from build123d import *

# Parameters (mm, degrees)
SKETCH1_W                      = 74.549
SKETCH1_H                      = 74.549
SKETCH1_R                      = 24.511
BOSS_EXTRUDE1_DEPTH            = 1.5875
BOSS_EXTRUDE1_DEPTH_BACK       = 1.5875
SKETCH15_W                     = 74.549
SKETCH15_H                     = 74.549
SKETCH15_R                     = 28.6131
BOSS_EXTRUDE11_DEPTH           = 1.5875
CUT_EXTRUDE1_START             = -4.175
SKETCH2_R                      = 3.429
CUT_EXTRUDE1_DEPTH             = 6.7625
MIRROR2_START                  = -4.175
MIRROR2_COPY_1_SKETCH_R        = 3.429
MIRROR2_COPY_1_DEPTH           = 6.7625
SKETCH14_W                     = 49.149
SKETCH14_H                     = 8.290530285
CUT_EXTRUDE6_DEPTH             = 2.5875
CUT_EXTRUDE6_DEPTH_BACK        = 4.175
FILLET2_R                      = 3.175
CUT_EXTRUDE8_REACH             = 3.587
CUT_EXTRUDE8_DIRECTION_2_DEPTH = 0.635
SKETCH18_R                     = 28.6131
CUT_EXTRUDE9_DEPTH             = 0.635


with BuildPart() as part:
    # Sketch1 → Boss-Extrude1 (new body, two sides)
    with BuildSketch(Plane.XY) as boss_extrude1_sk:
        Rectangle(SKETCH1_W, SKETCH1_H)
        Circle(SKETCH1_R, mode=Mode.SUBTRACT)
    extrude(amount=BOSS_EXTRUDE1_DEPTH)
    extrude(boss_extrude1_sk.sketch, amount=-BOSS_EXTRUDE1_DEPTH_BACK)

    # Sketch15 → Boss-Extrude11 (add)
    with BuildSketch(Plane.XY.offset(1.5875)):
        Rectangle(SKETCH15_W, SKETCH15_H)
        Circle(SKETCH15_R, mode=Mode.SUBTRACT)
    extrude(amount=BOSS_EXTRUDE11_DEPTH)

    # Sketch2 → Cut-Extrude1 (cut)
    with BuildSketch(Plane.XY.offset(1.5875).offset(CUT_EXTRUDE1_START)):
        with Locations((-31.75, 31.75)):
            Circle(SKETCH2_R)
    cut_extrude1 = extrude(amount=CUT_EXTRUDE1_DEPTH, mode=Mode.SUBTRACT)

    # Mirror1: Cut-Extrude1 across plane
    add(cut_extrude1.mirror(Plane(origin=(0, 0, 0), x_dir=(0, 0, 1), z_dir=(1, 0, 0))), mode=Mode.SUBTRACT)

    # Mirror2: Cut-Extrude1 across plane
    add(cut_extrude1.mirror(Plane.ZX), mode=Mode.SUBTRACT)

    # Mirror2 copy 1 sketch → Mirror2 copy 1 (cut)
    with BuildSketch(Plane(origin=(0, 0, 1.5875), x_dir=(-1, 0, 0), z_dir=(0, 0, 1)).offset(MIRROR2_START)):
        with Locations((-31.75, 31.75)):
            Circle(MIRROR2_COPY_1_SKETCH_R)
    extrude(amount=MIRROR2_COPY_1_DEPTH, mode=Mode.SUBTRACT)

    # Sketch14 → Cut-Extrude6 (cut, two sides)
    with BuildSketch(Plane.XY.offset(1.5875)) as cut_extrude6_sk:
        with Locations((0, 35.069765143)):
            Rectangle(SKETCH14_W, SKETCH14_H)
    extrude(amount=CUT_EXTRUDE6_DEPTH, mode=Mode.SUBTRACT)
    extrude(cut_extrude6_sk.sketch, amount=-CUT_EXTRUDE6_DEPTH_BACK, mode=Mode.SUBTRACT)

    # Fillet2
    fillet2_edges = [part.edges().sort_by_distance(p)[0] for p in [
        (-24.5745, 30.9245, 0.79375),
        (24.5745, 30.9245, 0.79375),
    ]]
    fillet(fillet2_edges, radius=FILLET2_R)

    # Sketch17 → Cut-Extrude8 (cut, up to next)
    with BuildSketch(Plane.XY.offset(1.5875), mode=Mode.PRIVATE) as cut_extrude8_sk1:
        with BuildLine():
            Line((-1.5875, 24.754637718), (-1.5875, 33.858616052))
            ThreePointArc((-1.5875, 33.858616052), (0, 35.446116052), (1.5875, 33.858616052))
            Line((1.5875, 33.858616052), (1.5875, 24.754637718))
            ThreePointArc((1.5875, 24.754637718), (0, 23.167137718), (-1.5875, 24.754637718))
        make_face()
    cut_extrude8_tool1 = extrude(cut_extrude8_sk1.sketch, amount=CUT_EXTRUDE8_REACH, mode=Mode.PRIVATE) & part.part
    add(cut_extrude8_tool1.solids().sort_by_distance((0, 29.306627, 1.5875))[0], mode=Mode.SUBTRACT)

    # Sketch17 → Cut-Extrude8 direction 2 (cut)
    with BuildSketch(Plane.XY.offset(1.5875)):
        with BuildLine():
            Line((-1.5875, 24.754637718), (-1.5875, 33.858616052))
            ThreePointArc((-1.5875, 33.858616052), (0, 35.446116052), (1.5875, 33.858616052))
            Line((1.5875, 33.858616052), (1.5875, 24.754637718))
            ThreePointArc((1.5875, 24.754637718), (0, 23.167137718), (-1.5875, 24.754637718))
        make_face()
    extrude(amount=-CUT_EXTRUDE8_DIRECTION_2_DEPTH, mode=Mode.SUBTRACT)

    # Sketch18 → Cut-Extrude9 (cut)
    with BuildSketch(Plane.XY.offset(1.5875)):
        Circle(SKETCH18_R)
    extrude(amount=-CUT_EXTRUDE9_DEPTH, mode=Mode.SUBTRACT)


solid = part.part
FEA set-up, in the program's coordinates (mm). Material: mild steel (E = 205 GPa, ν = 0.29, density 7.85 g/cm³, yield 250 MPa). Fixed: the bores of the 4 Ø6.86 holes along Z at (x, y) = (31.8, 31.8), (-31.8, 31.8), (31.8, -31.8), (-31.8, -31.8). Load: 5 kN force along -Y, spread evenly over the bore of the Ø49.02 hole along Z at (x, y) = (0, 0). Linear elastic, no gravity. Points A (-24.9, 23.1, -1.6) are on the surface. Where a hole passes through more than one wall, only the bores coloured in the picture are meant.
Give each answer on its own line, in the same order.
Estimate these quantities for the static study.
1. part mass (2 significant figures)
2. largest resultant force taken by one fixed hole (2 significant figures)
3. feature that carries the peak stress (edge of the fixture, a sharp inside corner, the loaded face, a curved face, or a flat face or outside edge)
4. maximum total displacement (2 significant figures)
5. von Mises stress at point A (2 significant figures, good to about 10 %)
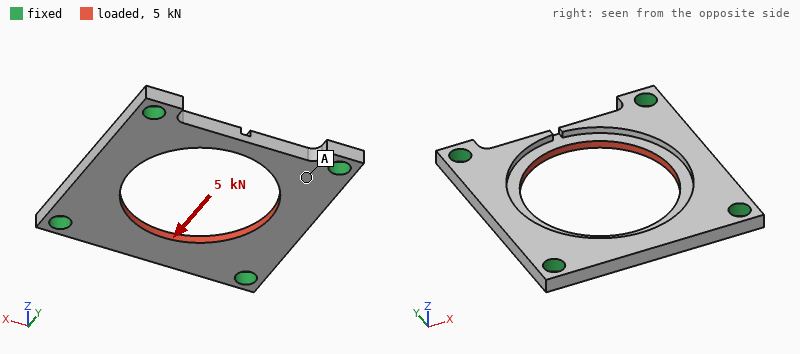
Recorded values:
110 g
1.3 kN
a flat face or outside edge
15 µm
16 MPa
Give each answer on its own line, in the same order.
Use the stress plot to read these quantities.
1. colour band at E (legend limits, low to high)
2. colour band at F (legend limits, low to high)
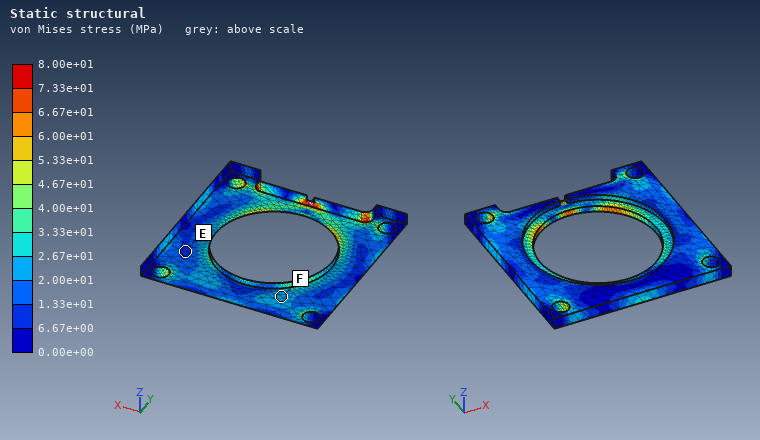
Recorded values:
6.67e+00 to 1.33e+01 MPa
2.00e+01 to 2.67e+01 MPa
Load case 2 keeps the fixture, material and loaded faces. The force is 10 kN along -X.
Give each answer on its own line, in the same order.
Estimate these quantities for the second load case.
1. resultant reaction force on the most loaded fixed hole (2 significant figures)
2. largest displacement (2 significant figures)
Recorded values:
2.7 kN
19 µm
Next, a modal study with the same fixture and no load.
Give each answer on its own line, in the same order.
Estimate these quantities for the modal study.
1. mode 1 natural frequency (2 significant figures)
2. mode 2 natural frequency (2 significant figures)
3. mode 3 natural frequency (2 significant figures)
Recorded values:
7200 Hz
7300 Hz
7300 Hz
